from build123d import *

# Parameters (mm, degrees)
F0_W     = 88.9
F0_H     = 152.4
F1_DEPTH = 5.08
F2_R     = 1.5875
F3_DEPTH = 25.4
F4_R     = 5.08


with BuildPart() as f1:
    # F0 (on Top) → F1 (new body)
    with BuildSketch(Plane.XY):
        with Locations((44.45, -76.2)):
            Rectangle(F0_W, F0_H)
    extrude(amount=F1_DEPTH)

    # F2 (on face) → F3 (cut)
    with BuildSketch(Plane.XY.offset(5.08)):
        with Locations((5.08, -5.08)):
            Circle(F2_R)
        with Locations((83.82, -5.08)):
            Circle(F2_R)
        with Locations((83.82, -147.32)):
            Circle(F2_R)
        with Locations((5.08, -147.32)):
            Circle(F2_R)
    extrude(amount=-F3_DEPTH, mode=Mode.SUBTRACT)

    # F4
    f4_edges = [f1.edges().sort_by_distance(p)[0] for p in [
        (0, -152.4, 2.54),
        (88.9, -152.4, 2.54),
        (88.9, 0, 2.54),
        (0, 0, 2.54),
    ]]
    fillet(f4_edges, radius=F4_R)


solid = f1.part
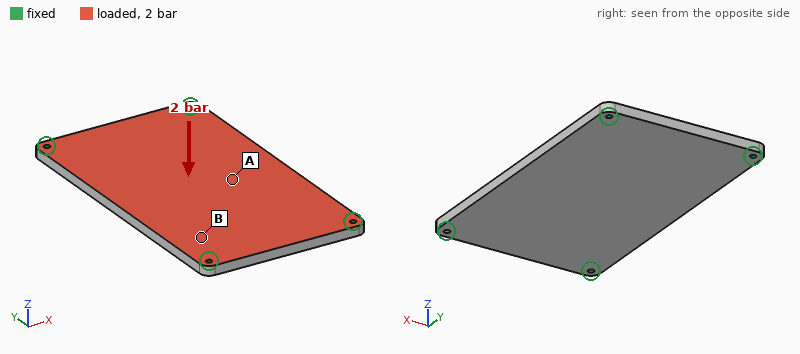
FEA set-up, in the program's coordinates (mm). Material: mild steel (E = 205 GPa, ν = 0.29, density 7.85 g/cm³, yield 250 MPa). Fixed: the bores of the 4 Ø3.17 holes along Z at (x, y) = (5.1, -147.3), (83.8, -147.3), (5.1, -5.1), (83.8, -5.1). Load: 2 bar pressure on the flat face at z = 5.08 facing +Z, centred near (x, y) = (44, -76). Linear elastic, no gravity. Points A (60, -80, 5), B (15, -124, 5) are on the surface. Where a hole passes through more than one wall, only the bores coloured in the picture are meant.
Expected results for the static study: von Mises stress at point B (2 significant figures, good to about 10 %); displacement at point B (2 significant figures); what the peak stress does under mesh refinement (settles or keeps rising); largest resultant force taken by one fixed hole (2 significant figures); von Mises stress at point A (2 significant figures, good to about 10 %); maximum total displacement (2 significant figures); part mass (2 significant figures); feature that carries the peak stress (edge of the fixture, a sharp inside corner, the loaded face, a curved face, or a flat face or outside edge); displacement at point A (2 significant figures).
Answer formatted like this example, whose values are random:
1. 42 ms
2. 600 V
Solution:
1. 16 MPa
2. 0.067 mm
3. keeps rising
4. 670 N
5. 47 MPa
6. 0.16 mm
7. 540 g
8. edge of the fixture
9. 0.16 mm
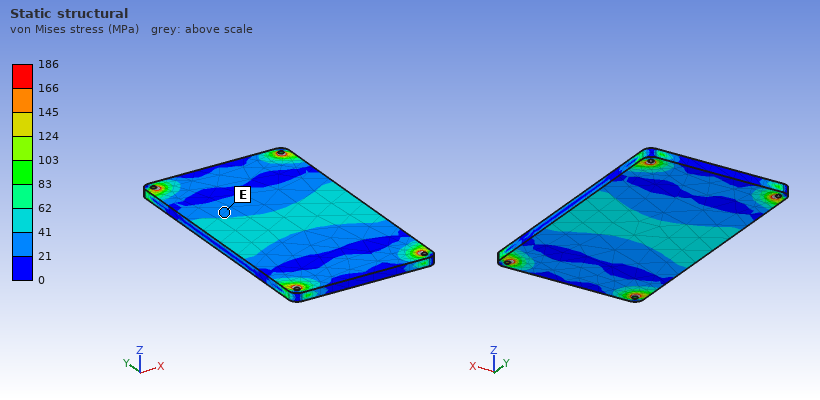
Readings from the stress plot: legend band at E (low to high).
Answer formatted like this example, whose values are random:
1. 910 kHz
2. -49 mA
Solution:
1. 21 to 41 MPa
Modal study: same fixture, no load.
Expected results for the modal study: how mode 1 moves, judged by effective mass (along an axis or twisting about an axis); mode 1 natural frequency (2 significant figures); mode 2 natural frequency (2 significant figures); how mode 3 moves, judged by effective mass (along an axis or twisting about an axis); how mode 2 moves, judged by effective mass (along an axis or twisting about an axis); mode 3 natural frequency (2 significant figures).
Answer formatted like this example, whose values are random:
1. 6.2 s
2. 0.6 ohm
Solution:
1. along Z
2. 1000 Hz
3. 1800 Hz
4. twisting about X
5. twisting about Y
6. 2700 Hz
